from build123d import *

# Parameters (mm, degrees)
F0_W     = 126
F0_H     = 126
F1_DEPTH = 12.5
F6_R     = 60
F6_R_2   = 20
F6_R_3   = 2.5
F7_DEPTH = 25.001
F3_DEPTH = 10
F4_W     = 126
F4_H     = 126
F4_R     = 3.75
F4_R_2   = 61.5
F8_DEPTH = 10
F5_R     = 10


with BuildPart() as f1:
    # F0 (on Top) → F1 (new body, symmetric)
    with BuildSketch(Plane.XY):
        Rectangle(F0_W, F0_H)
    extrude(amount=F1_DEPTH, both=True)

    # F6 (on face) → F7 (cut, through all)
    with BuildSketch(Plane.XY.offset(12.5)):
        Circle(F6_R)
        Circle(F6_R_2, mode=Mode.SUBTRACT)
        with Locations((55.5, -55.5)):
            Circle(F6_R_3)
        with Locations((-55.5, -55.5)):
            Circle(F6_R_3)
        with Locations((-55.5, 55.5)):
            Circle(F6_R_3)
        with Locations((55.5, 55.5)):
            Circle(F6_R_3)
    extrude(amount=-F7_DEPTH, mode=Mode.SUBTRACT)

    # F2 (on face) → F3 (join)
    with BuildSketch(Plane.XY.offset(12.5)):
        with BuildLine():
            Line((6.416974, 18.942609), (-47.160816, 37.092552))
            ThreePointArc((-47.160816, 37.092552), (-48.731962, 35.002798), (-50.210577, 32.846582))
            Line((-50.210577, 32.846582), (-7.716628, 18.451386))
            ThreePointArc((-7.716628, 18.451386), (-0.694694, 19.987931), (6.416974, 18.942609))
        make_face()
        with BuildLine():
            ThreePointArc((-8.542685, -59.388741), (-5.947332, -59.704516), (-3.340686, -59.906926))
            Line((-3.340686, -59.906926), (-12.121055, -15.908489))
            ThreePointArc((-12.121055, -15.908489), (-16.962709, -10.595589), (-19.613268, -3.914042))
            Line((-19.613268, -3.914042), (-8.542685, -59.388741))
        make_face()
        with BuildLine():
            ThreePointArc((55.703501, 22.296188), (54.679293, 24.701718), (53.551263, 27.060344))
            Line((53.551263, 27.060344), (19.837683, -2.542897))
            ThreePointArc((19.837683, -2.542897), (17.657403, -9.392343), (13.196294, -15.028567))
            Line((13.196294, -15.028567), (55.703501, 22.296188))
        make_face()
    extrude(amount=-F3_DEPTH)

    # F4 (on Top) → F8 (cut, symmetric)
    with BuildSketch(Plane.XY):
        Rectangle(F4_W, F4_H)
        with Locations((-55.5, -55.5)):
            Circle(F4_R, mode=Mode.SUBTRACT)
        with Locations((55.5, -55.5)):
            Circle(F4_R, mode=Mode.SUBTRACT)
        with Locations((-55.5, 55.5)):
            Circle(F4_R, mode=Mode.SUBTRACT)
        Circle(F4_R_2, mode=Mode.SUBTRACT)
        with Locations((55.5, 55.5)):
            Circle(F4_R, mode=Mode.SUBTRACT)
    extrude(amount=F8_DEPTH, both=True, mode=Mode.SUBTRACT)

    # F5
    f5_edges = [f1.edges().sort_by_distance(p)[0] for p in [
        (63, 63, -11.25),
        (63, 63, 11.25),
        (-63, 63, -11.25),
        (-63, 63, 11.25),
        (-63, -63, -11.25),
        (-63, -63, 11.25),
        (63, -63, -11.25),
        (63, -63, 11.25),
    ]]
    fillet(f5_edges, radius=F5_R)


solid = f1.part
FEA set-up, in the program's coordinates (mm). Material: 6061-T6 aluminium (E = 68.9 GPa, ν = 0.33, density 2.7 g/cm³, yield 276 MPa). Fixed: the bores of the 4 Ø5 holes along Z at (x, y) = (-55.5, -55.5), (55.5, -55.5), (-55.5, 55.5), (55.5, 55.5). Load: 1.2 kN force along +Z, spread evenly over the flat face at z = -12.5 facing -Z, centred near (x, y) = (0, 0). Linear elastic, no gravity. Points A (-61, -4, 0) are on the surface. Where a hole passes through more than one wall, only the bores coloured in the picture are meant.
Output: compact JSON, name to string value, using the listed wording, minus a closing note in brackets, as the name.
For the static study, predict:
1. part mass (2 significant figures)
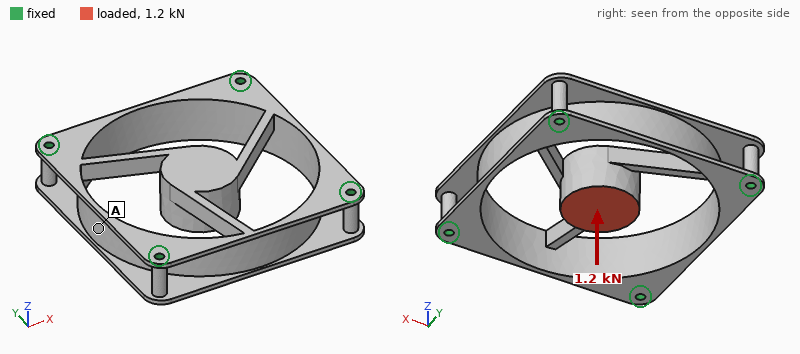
{"part mass": "200 g"}
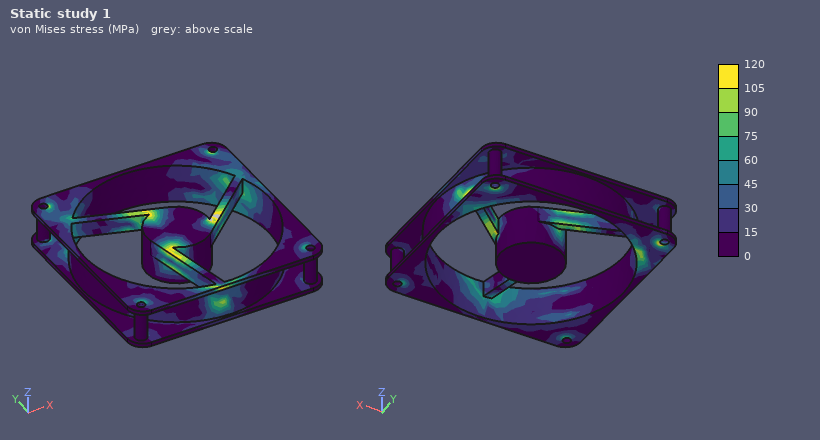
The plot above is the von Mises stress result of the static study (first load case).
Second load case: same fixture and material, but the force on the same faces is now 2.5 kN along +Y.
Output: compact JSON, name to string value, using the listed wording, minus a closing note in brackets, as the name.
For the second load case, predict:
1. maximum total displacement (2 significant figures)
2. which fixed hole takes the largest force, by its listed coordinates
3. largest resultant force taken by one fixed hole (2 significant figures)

{"maximum total displacement": "0.54 mm", "which fixed hole takes the largest force, by its listed coordinates": "(-55.5, -55.5)", "largest resultant force taken by one fixed hole": "2.0 kN"}
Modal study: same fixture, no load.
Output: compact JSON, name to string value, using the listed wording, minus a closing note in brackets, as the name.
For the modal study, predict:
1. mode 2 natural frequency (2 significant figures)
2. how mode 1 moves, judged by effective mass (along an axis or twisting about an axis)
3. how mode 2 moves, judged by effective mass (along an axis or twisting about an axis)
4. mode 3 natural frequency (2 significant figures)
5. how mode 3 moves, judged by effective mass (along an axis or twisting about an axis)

{"mode 2 natural frequency": "1500 Hz", "how mode 1 moves, judged by effective mass": "along Z", "how mode 2 moves, judged by effective mass": "along Y", "mode 3 natural frequency": "2100 Hz", "how mode 3 moves, judged by effective mass": "along X"}
